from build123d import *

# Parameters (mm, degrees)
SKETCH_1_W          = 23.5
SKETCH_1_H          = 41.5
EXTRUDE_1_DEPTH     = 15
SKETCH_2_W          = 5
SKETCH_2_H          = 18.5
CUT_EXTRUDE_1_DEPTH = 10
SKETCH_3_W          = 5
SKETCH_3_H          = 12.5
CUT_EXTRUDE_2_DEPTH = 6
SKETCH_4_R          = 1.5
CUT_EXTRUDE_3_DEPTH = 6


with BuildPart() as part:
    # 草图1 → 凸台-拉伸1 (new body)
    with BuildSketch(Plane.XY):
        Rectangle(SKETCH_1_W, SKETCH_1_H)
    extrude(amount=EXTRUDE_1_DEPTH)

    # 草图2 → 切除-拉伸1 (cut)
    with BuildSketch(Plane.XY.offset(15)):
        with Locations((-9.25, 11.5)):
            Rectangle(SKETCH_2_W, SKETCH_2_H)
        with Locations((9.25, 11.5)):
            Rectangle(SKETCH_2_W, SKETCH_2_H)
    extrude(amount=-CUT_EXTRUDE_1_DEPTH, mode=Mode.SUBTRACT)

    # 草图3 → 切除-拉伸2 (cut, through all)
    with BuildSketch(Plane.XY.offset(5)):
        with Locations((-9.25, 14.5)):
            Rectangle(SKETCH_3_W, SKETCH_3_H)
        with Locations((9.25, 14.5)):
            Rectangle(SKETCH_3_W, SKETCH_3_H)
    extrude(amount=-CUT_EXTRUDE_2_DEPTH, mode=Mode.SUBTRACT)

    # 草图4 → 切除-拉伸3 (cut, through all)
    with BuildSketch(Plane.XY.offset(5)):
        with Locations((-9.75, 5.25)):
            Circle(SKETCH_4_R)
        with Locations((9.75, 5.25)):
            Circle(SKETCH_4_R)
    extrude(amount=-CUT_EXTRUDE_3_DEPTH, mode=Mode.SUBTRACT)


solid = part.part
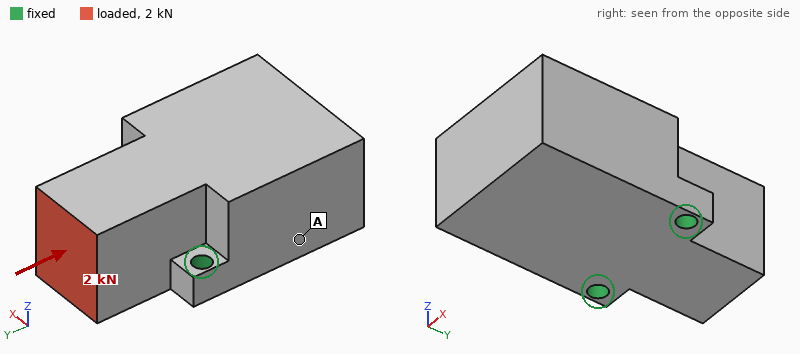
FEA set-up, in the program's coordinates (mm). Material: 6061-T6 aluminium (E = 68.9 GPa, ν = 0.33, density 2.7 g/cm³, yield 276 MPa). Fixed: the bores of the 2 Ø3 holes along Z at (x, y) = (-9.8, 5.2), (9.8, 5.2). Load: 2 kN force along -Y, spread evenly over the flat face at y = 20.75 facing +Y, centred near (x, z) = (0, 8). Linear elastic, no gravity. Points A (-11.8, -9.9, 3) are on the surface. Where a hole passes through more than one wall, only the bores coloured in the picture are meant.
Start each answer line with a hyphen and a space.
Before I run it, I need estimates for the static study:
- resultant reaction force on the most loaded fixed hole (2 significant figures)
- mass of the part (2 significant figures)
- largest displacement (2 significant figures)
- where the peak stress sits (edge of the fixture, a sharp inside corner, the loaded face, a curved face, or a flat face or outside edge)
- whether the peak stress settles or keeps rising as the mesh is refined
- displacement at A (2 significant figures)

- 1.0 kN
- 33 g
- 70 µm
- edge of the fixture
- keeps rising
- 34 µm
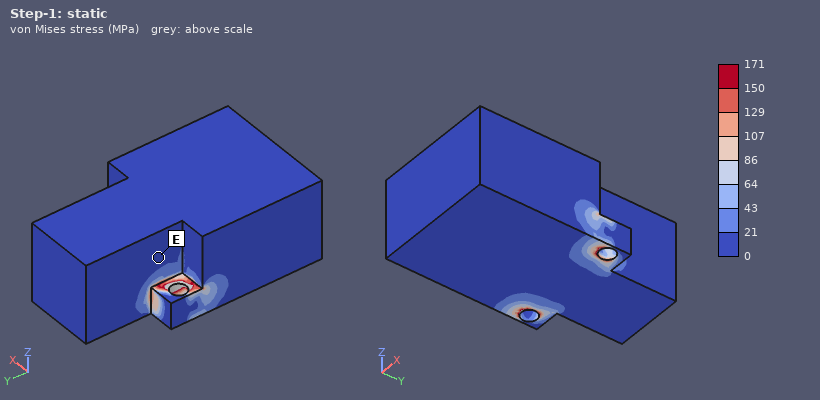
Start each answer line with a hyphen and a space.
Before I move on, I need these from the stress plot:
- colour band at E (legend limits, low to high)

- 0 to 21 MPa
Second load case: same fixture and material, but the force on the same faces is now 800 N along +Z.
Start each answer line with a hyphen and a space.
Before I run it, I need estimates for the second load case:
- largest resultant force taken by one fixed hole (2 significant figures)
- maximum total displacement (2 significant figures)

- 480 N
- 84 µm
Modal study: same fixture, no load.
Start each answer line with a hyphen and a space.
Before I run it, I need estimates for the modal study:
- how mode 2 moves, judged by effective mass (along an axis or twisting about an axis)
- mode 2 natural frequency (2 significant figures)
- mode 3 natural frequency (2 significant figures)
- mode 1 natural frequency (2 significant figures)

- along X
- 13 kHz
- 17 kHz
- 3800 Hz
